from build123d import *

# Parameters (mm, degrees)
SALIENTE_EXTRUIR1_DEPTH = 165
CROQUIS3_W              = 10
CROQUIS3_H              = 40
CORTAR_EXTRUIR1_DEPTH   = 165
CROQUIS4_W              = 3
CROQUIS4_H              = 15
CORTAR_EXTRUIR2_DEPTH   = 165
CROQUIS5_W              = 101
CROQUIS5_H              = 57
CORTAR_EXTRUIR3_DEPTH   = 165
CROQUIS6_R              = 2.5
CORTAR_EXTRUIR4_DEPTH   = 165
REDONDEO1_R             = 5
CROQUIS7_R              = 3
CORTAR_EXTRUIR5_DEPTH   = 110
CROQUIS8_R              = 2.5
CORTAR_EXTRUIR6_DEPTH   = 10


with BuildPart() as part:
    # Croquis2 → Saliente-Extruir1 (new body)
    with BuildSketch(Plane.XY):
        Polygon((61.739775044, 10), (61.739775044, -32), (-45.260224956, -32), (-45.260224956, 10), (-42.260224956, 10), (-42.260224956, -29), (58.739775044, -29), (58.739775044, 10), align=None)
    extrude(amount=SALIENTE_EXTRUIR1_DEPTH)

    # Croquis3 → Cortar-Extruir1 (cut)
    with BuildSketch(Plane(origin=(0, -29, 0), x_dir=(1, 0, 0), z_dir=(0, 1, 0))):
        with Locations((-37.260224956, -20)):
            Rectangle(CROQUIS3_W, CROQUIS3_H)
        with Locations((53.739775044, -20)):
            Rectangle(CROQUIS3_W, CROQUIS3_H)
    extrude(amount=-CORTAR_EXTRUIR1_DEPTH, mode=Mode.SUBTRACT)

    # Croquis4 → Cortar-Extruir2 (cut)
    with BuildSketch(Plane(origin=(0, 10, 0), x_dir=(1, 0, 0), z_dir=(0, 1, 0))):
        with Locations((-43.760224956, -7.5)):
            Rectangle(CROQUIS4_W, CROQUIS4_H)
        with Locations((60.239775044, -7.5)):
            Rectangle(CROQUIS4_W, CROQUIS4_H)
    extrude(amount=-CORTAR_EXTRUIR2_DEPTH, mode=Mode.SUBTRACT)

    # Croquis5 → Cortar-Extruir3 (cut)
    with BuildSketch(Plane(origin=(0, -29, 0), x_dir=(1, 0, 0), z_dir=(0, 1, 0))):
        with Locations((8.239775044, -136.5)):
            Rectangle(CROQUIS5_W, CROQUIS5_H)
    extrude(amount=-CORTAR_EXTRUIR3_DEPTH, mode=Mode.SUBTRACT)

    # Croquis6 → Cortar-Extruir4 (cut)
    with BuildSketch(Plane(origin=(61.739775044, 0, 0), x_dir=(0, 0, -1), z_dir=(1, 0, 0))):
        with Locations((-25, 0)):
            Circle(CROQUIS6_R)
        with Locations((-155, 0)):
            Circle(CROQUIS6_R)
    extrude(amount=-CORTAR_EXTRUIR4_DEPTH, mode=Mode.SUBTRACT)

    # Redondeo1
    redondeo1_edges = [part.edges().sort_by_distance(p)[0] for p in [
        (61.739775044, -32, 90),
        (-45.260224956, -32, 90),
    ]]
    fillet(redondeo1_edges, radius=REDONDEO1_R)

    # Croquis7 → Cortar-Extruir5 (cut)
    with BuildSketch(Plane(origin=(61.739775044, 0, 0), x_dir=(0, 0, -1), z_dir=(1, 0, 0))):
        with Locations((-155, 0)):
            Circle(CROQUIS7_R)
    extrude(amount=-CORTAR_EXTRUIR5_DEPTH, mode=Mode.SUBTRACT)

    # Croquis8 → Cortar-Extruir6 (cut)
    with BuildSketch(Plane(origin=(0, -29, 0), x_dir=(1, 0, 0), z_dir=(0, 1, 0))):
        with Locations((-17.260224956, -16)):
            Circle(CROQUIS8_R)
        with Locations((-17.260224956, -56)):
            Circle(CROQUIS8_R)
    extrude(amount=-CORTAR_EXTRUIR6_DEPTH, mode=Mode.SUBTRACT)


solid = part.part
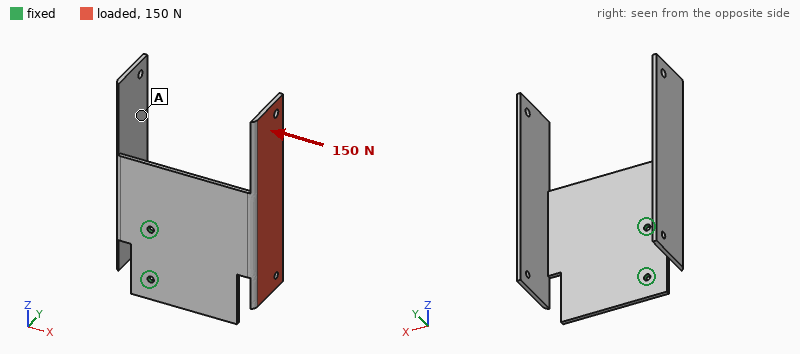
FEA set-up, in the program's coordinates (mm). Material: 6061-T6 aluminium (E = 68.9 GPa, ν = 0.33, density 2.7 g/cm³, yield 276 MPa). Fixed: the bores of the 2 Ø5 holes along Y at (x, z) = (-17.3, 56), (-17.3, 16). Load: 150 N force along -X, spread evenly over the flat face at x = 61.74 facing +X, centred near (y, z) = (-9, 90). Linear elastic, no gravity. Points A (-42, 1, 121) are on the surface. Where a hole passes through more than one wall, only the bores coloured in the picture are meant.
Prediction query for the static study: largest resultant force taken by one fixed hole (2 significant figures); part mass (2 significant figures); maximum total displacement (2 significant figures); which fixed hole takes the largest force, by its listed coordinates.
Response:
270 N
180 g
1.9 mm
(-17.3, 56)
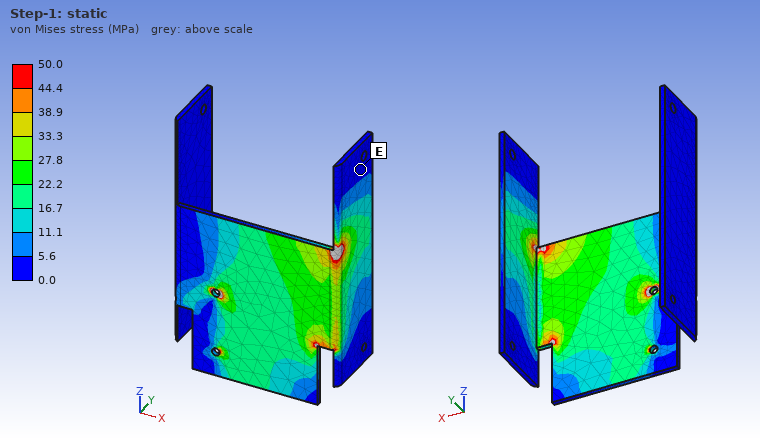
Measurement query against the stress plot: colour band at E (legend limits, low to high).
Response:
0.0 to 5.6 MPa
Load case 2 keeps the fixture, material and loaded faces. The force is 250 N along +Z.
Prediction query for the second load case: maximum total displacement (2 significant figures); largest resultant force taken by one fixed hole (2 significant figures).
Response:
2.2 mm
490 N
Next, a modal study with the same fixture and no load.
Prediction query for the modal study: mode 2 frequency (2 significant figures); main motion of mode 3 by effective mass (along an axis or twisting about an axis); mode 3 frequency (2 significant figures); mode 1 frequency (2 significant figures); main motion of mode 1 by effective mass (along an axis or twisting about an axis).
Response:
260 Hz
along Y
310 Hz
150 Hz
along Y
